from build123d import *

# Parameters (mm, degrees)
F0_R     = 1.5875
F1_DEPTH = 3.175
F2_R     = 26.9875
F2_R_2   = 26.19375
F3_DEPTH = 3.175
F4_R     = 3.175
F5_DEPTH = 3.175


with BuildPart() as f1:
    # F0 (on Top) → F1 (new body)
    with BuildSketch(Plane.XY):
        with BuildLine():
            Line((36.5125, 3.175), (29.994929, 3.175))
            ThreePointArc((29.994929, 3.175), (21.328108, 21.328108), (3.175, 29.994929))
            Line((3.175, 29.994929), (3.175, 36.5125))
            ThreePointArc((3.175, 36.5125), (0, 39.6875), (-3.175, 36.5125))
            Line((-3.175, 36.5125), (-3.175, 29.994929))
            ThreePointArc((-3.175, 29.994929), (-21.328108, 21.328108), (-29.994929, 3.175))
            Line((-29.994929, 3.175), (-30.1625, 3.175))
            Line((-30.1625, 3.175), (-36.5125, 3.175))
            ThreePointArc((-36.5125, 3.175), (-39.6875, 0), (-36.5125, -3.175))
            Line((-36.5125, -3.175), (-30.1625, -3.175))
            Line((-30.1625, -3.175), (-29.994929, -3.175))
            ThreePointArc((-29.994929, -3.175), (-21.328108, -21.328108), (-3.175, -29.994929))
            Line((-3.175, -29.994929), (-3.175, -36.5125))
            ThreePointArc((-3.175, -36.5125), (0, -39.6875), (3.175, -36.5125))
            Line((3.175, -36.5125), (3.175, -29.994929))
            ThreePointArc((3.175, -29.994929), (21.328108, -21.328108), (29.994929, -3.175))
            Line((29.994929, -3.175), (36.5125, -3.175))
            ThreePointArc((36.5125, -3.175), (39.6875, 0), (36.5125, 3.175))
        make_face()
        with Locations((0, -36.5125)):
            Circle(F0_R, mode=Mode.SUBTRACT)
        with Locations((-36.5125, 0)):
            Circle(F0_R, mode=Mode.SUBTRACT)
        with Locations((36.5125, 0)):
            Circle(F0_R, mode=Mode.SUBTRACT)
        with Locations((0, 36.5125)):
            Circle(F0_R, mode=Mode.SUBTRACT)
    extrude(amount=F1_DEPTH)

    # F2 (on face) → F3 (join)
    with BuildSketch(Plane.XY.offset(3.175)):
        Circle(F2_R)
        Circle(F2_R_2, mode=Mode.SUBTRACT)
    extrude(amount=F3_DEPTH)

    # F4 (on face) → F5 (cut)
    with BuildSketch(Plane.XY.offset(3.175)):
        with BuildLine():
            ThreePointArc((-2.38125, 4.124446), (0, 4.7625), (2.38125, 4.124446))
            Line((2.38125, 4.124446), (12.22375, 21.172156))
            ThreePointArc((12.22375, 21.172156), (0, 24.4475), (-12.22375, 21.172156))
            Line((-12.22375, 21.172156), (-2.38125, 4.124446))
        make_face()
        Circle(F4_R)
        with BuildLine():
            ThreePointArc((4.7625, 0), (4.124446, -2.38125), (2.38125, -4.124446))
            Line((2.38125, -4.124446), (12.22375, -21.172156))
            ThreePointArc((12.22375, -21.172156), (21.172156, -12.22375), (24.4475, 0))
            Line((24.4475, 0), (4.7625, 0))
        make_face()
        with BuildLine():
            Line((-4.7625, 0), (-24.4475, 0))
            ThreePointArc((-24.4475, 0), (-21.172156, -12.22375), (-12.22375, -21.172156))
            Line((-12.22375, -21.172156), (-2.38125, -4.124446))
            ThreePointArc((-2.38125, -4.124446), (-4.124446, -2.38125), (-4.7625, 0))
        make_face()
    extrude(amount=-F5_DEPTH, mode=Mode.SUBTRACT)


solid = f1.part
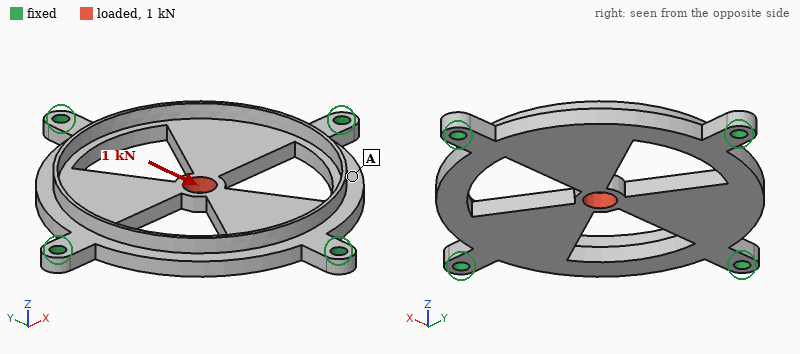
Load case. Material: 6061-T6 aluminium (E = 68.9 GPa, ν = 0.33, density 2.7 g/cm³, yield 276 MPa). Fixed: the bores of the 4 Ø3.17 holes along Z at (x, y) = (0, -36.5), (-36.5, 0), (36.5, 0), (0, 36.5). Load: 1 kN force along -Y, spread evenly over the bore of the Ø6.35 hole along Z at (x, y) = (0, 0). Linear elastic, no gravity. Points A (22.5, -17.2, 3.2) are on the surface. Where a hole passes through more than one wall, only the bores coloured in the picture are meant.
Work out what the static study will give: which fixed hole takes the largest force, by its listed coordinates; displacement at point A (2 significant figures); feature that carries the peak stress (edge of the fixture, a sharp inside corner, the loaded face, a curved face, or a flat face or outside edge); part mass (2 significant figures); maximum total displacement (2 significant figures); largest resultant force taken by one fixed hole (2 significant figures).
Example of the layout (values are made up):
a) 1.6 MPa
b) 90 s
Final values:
a) (0, -36.5)
b) 5.1 µm
c) the loaded face
d) 19 g
e) 24 µm
f) 630 N
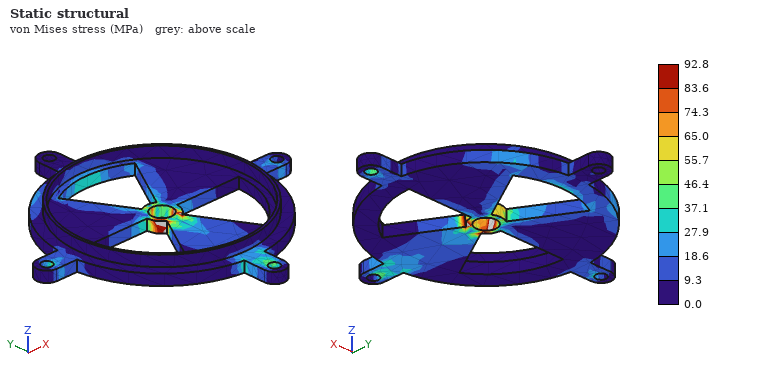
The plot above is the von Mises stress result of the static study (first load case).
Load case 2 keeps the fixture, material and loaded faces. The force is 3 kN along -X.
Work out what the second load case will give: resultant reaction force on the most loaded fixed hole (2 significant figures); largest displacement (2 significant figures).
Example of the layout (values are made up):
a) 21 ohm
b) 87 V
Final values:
a) 1.1 kN
b) 82 µm
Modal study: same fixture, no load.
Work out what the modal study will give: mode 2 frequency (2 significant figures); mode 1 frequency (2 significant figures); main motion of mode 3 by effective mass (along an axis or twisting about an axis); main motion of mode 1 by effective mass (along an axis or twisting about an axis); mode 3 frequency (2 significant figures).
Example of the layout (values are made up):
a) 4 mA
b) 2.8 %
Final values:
a) 5400 Hz
b) 3700 Hz
c) twisting about X
d) along Z
e) 5900 Hz
